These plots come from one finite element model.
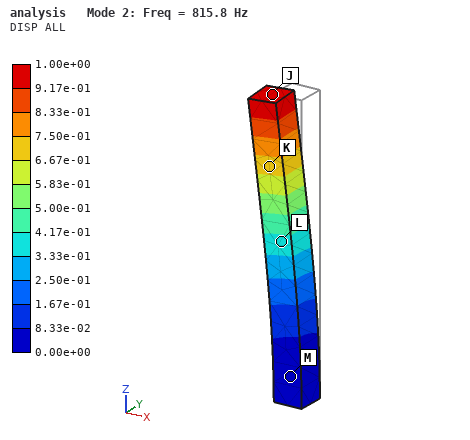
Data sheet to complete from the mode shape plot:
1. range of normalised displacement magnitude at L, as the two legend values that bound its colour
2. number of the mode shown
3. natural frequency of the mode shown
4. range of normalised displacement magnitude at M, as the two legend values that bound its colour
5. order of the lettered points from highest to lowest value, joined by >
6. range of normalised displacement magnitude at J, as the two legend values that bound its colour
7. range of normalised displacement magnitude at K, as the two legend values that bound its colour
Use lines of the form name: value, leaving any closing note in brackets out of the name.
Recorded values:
range of normalised displacement magnitude at L, as the two legend values that bound its colour: 3.33e-01 to 4.17e-01
number of the mode shown: 2
natural frequency of the mode shown: 815.8 Hz
range of normalised displacement magnitude at M, as the two legend values that bound its colour: 0.00e+00 to 8.33e-02
order of the lettered points from highest to lowest value, joined by >: J > K > L > M
range of normalised displacement magnitude at J, as the two legend values that bound its colour: 9.17e-01 to 1.00e+00
range of normalised displacement magnitude at K, as the two legend values that bound its colour: 6.67e-01 to 7.50e-01
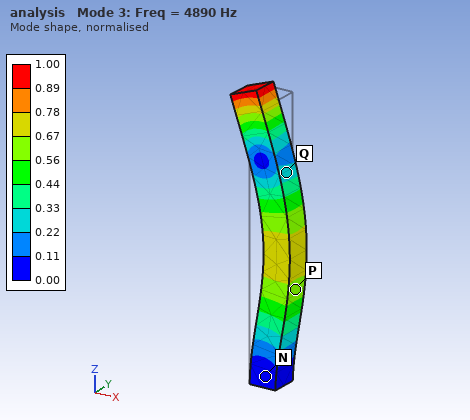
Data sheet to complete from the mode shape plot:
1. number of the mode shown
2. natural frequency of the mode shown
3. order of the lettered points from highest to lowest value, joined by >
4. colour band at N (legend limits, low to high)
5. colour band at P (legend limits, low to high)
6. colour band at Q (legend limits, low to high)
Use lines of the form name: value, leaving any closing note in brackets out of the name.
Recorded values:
number of the mode shown: 3
natural frequency of the mode shown: 4890 Hz
order of the lettered points from highest to lowest value, joined by >: P > Q > N
colour band at N: 0.00 to 0.11
colour band at P: 0.56 to 0.67
colour band at Q: 0.22 to 0.33
